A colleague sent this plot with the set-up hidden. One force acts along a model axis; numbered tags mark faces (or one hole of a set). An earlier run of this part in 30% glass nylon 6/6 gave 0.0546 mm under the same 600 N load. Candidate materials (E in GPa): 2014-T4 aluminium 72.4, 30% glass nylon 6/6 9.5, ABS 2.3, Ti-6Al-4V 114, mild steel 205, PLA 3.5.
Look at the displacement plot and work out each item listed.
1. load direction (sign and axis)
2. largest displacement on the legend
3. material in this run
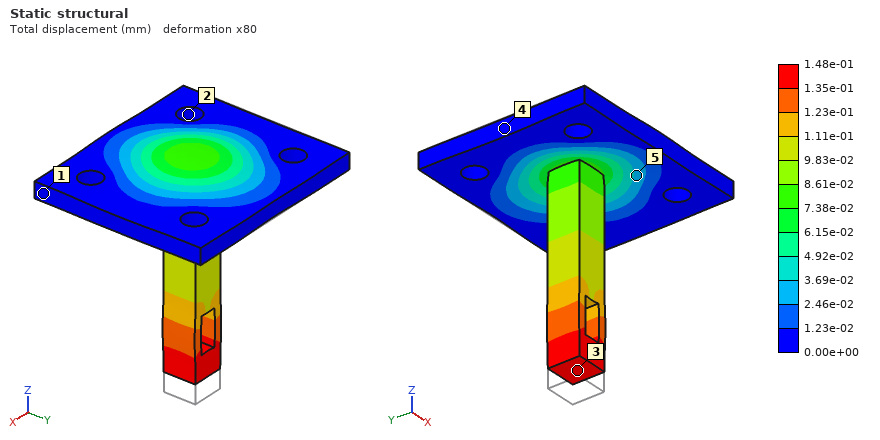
+Z
1.48e-01 mm
PLA
